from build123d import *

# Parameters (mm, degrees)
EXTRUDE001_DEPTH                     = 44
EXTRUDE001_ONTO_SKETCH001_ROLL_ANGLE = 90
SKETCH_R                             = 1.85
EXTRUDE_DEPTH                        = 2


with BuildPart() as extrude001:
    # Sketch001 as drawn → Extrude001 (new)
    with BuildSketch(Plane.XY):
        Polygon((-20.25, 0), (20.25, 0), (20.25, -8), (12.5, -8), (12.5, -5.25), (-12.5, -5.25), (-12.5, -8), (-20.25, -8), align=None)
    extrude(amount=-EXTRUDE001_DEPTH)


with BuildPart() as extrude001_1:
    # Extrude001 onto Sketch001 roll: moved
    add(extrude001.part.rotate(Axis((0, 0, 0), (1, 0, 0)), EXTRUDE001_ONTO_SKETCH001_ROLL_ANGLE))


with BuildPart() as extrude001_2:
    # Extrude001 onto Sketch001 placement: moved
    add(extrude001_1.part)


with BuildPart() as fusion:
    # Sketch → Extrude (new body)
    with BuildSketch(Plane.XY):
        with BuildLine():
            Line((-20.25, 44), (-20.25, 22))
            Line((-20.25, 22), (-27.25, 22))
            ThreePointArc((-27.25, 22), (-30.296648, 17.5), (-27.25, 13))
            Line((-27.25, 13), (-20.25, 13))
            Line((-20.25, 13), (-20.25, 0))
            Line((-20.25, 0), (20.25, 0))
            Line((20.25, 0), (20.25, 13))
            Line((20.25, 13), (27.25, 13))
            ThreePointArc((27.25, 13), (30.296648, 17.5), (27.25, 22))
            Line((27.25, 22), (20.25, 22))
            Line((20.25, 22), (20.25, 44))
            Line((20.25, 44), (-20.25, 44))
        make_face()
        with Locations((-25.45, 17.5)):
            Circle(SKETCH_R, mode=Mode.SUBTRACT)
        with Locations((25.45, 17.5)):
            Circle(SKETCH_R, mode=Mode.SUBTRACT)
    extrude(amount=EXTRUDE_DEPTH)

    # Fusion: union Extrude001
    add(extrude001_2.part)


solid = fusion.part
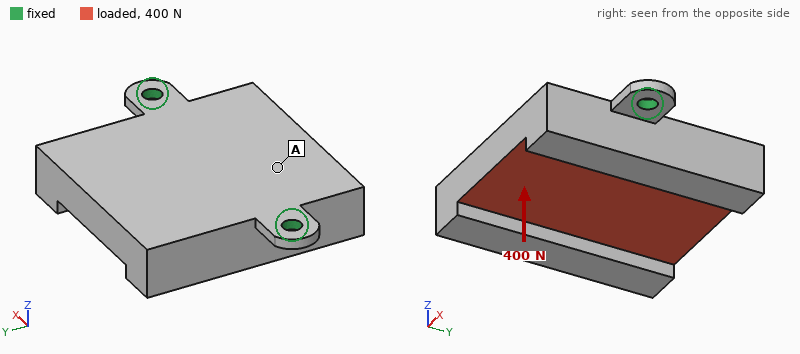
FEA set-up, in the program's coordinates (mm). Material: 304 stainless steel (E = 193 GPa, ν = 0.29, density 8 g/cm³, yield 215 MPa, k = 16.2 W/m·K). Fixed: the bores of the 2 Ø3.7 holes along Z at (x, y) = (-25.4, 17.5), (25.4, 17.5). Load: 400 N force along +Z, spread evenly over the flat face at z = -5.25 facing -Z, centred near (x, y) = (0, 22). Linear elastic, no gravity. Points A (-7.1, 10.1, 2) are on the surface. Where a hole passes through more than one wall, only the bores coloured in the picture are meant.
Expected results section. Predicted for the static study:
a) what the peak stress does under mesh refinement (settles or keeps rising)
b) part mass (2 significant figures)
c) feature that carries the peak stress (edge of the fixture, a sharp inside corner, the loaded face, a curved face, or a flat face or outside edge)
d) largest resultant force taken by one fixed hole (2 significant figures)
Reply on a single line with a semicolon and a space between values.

keeps rising; 120 g; edge of the fixture; 280 N
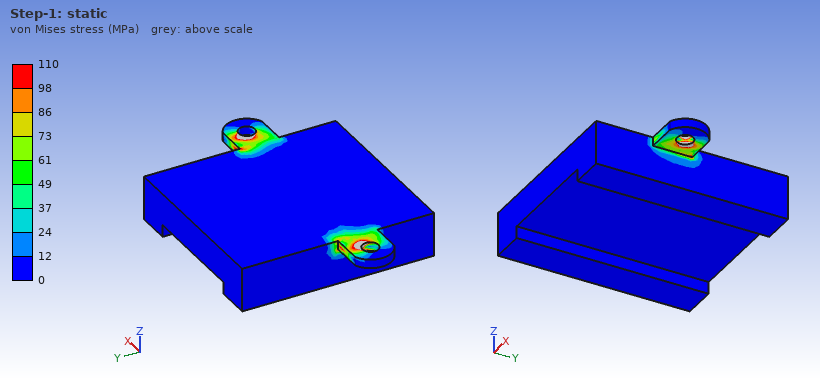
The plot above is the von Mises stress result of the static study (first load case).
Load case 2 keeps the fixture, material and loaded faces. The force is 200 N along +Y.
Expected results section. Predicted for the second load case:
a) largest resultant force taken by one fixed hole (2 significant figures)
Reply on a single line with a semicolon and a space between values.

100 N
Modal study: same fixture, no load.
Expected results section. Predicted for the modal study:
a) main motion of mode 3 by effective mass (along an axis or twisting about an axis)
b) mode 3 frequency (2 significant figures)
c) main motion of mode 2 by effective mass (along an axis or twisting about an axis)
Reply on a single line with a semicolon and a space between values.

twisting about Y; 7900 Hz; along Z
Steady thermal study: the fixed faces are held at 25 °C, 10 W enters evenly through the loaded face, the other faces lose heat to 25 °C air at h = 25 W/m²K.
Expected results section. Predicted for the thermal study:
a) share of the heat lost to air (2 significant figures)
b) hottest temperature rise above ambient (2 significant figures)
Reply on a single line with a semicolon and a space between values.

55 %; 60 K
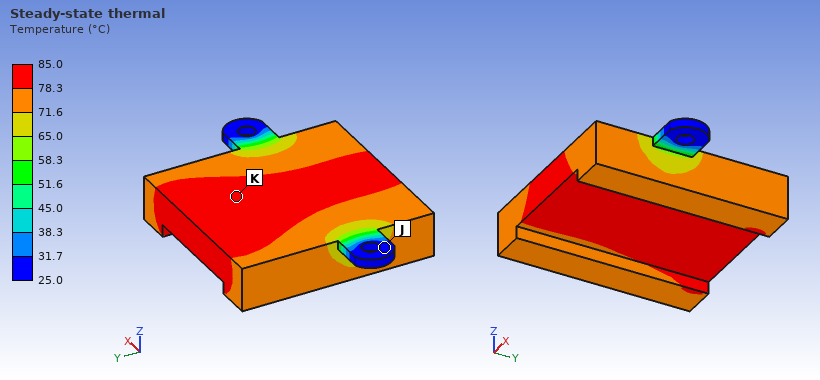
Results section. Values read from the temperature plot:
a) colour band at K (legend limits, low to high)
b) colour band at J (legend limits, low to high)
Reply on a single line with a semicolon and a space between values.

78.3 to 85.0 °C; 25.0 to 31.7 °C
